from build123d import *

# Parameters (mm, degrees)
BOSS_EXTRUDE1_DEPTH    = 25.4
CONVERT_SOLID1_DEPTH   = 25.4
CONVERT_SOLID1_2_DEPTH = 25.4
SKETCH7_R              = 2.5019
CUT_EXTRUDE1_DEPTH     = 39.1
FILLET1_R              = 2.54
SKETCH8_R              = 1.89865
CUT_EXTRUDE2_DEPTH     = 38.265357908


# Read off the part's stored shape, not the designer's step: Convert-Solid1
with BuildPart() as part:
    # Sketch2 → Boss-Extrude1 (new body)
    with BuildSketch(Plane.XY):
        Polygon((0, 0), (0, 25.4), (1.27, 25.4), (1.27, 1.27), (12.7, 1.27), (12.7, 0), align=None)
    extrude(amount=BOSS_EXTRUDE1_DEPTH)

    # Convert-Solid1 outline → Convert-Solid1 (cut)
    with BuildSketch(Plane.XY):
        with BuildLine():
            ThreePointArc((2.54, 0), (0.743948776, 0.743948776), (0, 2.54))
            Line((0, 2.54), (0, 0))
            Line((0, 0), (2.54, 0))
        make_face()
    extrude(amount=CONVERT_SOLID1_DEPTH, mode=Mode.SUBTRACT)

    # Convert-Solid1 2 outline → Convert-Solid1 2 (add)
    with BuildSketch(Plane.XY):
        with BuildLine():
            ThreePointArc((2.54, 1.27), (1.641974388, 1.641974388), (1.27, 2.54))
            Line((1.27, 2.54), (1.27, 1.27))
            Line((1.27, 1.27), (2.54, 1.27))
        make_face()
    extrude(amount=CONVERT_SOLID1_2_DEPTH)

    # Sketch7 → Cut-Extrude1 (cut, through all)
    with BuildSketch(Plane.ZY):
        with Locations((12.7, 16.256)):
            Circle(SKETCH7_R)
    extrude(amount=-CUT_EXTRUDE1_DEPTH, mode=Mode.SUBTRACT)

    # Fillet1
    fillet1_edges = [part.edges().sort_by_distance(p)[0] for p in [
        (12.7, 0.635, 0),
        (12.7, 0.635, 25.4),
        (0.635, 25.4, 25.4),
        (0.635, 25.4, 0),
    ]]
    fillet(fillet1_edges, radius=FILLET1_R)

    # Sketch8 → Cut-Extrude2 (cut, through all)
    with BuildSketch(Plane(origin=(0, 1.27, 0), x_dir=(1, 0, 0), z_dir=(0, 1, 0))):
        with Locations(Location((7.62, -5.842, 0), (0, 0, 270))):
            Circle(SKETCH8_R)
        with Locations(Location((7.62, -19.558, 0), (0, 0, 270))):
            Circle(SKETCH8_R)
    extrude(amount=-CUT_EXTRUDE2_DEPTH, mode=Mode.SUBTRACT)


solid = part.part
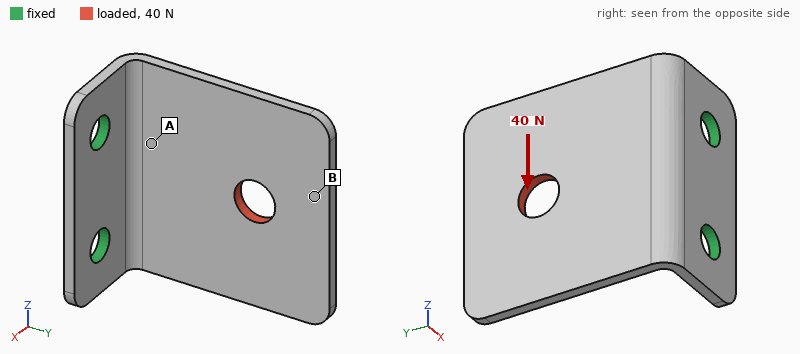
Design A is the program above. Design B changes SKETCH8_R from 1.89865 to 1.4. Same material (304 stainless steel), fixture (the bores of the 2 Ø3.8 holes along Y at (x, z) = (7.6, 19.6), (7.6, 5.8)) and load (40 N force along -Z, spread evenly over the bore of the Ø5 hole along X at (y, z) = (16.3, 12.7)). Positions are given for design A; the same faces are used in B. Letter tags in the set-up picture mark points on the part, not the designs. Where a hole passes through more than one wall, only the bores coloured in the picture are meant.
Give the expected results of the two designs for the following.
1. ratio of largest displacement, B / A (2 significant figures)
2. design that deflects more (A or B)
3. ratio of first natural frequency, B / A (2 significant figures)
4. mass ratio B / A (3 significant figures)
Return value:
1.2
B
0.97
1.01
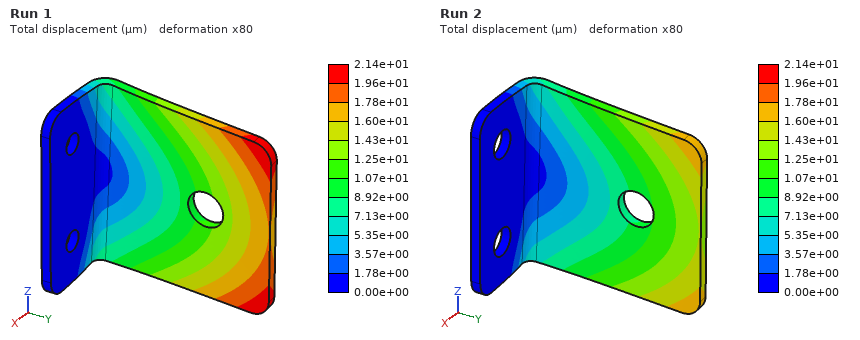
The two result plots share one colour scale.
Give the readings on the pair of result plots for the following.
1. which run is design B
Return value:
Run 1
